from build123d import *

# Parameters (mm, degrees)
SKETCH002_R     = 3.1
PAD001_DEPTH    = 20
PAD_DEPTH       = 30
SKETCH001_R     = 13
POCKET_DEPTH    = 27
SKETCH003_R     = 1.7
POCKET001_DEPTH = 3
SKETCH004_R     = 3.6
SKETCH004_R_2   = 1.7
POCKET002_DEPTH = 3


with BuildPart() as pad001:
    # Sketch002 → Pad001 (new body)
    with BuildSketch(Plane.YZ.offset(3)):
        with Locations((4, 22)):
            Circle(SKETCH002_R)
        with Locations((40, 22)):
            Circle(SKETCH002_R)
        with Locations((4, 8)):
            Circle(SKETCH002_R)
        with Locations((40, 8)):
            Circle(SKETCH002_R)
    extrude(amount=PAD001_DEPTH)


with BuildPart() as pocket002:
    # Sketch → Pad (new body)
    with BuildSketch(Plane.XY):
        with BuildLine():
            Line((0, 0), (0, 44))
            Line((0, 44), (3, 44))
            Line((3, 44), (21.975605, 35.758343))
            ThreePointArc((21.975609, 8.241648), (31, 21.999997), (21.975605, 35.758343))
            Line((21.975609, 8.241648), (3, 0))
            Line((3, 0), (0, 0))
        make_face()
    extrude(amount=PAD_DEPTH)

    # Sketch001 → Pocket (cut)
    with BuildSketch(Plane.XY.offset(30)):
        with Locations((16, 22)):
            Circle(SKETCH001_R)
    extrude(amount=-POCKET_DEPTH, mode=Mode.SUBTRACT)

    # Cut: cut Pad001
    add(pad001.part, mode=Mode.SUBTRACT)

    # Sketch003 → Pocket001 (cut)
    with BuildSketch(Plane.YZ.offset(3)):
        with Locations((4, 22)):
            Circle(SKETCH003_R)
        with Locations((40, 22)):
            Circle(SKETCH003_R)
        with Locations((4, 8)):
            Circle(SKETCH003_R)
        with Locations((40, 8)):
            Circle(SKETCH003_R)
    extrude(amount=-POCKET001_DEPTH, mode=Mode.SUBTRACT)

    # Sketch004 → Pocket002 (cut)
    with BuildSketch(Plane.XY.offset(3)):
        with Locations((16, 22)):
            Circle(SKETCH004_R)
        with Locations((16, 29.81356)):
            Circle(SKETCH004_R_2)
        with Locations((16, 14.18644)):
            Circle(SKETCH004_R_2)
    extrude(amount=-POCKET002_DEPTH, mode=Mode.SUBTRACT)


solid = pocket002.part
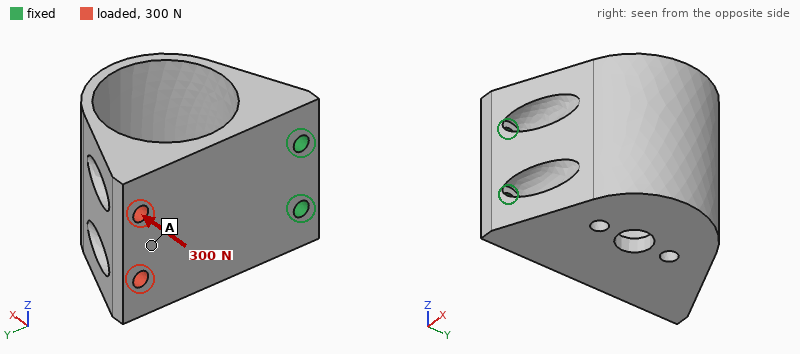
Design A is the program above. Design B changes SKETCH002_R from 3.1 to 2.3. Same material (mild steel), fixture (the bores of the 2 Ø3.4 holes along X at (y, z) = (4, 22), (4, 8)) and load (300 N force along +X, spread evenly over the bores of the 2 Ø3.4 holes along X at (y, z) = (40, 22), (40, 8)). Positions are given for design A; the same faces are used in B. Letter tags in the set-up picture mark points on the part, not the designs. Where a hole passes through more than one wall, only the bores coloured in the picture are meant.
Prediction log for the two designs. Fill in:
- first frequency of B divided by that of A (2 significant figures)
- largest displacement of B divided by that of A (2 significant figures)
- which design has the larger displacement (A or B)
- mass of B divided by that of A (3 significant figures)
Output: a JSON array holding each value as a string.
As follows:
["1.0", "0.89", "A", "1.04"]
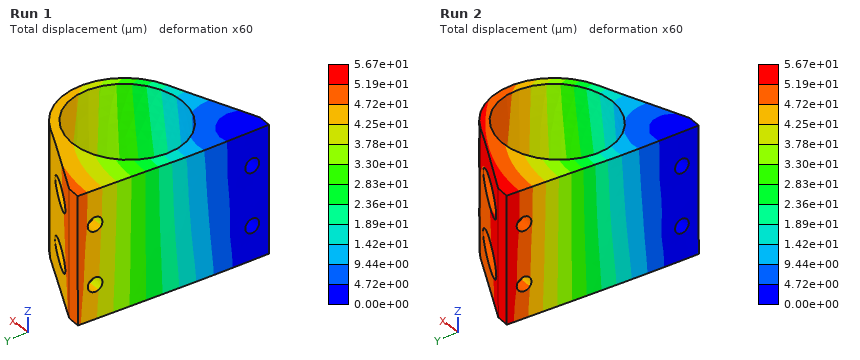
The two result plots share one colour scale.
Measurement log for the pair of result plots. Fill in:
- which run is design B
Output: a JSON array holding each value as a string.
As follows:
["Run 1"]
